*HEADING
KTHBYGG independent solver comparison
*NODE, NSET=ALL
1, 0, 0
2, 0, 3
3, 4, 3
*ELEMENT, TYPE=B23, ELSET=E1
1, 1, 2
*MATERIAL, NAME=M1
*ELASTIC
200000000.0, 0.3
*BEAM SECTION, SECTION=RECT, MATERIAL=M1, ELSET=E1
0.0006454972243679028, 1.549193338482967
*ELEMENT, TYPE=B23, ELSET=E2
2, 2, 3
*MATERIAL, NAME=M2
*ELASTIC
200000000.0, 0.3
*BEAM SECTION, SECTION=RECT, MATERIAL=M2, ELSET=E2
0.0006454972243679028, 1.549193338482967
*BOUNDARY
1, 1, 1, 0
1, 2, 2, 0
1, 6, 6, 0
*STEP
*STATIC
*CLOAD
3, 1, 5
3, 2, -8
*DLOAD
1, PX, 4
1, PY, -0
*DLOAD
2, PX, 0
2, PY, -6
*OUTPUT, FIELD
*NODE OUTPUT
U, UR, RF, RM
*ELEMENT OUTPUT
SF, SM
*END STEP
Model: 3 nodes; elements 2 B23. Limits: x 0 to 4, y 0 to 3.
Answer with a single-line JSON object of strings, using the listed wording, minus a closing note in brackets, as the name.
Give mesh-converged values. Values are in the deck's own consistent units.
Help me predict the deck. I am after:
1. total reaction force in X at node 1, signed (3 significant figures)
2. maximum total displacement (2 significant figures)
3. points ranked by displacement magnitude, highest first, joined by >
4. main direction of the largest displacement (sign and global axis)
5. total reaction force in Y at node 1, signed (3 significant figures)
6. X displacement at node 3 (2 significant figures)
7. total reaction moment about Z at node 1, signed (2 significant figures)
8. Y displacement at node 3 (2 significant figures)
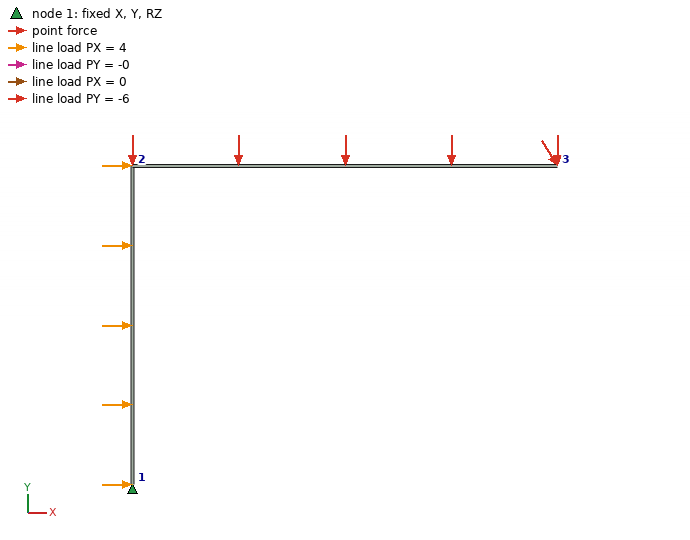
{"total reaction force in X at node 1, signed": "-17.0", "maximum total displacement": "0.039", "points ranked by displacement magnitude, highest first, joined by >": "node 3 > node 2 > node 1", "main direction of the largest displacement": "-Y", "total reaction force in Y at node 1, signed": "32.0", "X displacement at node 3": "0.011", "total reaction moment about Z at node 1, signed": "110", "Y displacement at node 3": "-0.038"}
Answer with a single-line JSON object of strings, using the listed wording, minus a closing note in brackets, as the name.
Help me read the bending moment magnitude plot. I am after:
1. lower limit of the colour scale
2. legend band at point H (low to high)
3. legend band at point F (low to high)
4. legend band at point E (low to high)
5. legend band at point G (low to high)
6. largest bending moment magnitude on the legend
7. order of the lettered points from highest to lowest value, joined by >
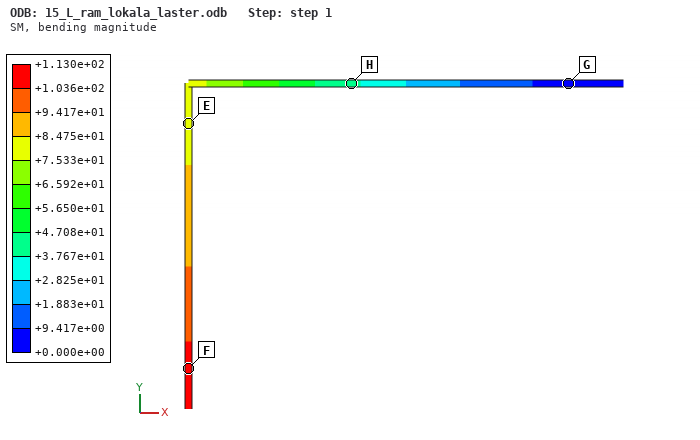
{"lower limit of the colour scale": "+0.000e+00", "legend band at point H": "+3.767e+01 to +4.708e+01", "legend band at point F": "+1.036e+02 to +1.130e+02", "legend band at point E": "+7.533e+01 to +8.475e+01", "legend band at point G": "+0.000e+00 to +9.417e+00", "largest bending moment magnitude on the legend": "+1.130e+02", "order of the lettered points from highest to lowest value, joined by >": "F > E > H > G"}
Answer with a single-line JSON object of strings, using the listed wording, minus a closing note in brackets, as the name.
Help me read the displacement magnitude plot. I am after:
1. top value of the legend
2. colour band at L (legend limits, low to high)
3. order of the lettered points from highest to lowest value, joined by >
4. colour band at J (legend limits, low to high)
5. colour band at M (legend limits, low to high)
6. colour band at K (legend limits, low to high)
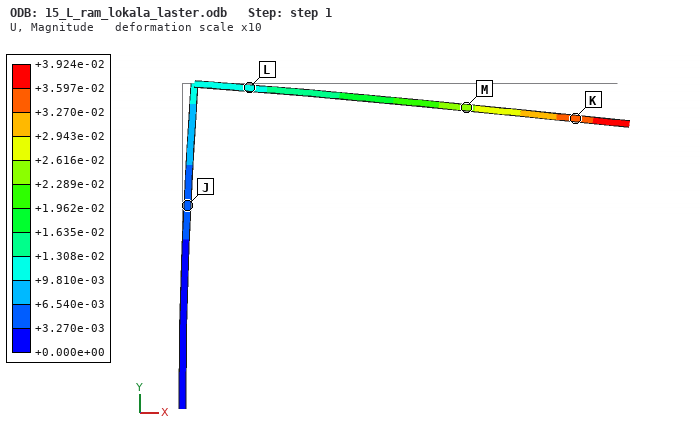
{"top value of the legend": "+3.924e-02", "colour band at L": "+9.810e-03 to +1.308e-02", "order of the lettered points from highest to lowest value, joined by >": "K > M > L > J", "colour band at J": "+3.270e-03 to +6.540e-03", "colour band at M": "+2.289e-02 to +2.616e-02", "colour band at K": "+3.270e-02 to +3.597e-02"}
